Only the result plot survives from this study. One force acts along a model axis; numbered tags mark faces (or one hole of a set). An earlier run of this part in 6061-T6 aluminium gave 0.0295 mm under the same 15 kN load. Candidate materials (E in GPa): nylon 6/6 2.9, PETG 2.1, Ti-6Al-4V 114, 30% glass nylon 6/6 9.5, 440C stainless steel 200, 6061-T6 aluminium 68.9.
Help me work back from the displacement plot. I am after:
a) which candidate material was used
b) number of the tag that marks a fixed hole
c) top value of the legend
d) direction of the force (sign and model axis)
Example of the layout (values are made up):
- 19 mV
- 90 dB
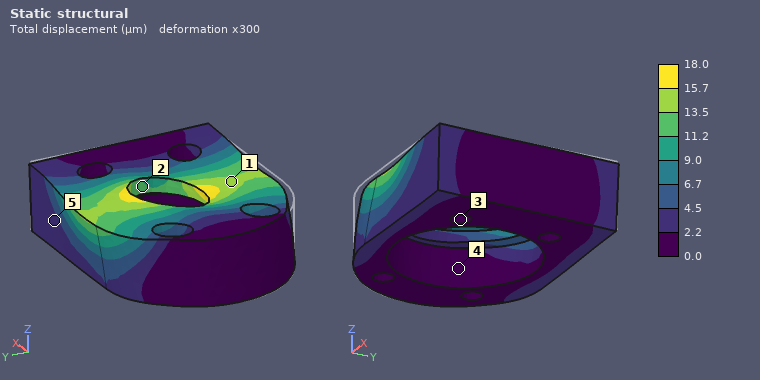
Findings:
- Ti-6Al-4V
- 3
- 18.0 µm
- +Y
